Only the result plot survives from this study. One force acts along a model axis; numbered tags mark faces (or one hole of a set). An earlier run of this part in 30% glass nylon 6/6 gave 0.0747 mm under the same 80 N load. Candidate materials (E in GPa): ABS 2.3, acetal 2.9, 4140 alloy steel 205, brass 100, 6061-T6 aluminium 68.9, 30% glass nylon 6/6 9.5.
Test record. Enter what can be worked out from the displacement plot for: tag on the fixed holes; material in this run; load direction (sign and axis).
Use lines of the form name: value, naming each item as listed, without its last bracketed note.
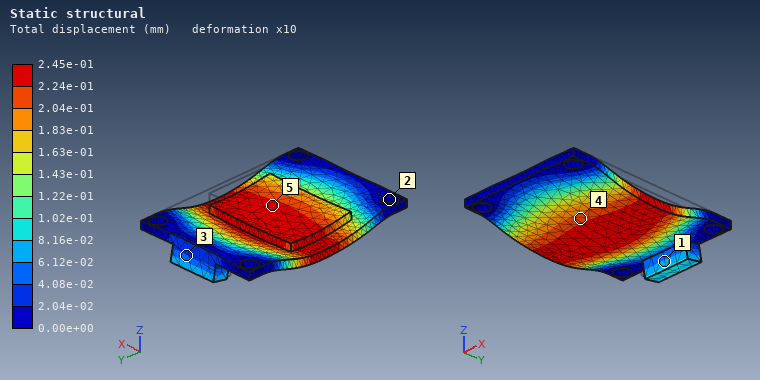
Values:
tag on the fixed holes: 2
material in this run: acetal
load direction: -Z
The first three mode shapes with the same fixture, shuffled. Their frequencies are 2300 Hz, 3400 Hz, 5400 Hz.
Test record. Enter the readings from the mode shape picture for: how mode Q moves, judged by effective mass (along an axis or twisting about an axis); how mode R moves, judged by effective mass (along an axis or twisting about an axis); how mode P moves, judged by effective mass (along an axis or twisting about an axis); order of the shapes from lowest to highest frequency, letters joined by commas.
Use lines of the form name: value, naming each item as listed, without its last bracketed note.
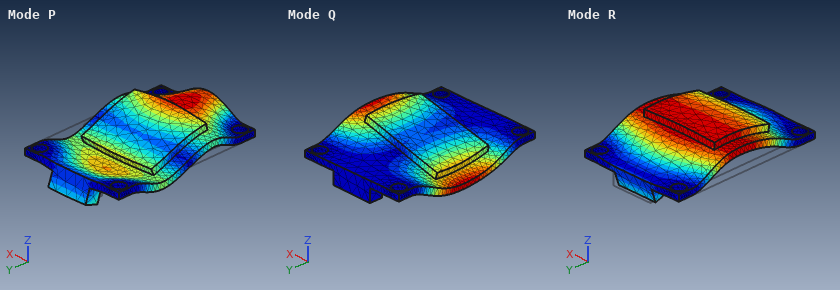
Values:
how mode Q moves, judged by effective mass: twisting about Y
how mode R moves, judged by effective mass: along Z
how mode P moves, judged by effective mass: twisting about X
order of the shapes from lowest to highest frequency, letters joined by commas: R, Q, P
